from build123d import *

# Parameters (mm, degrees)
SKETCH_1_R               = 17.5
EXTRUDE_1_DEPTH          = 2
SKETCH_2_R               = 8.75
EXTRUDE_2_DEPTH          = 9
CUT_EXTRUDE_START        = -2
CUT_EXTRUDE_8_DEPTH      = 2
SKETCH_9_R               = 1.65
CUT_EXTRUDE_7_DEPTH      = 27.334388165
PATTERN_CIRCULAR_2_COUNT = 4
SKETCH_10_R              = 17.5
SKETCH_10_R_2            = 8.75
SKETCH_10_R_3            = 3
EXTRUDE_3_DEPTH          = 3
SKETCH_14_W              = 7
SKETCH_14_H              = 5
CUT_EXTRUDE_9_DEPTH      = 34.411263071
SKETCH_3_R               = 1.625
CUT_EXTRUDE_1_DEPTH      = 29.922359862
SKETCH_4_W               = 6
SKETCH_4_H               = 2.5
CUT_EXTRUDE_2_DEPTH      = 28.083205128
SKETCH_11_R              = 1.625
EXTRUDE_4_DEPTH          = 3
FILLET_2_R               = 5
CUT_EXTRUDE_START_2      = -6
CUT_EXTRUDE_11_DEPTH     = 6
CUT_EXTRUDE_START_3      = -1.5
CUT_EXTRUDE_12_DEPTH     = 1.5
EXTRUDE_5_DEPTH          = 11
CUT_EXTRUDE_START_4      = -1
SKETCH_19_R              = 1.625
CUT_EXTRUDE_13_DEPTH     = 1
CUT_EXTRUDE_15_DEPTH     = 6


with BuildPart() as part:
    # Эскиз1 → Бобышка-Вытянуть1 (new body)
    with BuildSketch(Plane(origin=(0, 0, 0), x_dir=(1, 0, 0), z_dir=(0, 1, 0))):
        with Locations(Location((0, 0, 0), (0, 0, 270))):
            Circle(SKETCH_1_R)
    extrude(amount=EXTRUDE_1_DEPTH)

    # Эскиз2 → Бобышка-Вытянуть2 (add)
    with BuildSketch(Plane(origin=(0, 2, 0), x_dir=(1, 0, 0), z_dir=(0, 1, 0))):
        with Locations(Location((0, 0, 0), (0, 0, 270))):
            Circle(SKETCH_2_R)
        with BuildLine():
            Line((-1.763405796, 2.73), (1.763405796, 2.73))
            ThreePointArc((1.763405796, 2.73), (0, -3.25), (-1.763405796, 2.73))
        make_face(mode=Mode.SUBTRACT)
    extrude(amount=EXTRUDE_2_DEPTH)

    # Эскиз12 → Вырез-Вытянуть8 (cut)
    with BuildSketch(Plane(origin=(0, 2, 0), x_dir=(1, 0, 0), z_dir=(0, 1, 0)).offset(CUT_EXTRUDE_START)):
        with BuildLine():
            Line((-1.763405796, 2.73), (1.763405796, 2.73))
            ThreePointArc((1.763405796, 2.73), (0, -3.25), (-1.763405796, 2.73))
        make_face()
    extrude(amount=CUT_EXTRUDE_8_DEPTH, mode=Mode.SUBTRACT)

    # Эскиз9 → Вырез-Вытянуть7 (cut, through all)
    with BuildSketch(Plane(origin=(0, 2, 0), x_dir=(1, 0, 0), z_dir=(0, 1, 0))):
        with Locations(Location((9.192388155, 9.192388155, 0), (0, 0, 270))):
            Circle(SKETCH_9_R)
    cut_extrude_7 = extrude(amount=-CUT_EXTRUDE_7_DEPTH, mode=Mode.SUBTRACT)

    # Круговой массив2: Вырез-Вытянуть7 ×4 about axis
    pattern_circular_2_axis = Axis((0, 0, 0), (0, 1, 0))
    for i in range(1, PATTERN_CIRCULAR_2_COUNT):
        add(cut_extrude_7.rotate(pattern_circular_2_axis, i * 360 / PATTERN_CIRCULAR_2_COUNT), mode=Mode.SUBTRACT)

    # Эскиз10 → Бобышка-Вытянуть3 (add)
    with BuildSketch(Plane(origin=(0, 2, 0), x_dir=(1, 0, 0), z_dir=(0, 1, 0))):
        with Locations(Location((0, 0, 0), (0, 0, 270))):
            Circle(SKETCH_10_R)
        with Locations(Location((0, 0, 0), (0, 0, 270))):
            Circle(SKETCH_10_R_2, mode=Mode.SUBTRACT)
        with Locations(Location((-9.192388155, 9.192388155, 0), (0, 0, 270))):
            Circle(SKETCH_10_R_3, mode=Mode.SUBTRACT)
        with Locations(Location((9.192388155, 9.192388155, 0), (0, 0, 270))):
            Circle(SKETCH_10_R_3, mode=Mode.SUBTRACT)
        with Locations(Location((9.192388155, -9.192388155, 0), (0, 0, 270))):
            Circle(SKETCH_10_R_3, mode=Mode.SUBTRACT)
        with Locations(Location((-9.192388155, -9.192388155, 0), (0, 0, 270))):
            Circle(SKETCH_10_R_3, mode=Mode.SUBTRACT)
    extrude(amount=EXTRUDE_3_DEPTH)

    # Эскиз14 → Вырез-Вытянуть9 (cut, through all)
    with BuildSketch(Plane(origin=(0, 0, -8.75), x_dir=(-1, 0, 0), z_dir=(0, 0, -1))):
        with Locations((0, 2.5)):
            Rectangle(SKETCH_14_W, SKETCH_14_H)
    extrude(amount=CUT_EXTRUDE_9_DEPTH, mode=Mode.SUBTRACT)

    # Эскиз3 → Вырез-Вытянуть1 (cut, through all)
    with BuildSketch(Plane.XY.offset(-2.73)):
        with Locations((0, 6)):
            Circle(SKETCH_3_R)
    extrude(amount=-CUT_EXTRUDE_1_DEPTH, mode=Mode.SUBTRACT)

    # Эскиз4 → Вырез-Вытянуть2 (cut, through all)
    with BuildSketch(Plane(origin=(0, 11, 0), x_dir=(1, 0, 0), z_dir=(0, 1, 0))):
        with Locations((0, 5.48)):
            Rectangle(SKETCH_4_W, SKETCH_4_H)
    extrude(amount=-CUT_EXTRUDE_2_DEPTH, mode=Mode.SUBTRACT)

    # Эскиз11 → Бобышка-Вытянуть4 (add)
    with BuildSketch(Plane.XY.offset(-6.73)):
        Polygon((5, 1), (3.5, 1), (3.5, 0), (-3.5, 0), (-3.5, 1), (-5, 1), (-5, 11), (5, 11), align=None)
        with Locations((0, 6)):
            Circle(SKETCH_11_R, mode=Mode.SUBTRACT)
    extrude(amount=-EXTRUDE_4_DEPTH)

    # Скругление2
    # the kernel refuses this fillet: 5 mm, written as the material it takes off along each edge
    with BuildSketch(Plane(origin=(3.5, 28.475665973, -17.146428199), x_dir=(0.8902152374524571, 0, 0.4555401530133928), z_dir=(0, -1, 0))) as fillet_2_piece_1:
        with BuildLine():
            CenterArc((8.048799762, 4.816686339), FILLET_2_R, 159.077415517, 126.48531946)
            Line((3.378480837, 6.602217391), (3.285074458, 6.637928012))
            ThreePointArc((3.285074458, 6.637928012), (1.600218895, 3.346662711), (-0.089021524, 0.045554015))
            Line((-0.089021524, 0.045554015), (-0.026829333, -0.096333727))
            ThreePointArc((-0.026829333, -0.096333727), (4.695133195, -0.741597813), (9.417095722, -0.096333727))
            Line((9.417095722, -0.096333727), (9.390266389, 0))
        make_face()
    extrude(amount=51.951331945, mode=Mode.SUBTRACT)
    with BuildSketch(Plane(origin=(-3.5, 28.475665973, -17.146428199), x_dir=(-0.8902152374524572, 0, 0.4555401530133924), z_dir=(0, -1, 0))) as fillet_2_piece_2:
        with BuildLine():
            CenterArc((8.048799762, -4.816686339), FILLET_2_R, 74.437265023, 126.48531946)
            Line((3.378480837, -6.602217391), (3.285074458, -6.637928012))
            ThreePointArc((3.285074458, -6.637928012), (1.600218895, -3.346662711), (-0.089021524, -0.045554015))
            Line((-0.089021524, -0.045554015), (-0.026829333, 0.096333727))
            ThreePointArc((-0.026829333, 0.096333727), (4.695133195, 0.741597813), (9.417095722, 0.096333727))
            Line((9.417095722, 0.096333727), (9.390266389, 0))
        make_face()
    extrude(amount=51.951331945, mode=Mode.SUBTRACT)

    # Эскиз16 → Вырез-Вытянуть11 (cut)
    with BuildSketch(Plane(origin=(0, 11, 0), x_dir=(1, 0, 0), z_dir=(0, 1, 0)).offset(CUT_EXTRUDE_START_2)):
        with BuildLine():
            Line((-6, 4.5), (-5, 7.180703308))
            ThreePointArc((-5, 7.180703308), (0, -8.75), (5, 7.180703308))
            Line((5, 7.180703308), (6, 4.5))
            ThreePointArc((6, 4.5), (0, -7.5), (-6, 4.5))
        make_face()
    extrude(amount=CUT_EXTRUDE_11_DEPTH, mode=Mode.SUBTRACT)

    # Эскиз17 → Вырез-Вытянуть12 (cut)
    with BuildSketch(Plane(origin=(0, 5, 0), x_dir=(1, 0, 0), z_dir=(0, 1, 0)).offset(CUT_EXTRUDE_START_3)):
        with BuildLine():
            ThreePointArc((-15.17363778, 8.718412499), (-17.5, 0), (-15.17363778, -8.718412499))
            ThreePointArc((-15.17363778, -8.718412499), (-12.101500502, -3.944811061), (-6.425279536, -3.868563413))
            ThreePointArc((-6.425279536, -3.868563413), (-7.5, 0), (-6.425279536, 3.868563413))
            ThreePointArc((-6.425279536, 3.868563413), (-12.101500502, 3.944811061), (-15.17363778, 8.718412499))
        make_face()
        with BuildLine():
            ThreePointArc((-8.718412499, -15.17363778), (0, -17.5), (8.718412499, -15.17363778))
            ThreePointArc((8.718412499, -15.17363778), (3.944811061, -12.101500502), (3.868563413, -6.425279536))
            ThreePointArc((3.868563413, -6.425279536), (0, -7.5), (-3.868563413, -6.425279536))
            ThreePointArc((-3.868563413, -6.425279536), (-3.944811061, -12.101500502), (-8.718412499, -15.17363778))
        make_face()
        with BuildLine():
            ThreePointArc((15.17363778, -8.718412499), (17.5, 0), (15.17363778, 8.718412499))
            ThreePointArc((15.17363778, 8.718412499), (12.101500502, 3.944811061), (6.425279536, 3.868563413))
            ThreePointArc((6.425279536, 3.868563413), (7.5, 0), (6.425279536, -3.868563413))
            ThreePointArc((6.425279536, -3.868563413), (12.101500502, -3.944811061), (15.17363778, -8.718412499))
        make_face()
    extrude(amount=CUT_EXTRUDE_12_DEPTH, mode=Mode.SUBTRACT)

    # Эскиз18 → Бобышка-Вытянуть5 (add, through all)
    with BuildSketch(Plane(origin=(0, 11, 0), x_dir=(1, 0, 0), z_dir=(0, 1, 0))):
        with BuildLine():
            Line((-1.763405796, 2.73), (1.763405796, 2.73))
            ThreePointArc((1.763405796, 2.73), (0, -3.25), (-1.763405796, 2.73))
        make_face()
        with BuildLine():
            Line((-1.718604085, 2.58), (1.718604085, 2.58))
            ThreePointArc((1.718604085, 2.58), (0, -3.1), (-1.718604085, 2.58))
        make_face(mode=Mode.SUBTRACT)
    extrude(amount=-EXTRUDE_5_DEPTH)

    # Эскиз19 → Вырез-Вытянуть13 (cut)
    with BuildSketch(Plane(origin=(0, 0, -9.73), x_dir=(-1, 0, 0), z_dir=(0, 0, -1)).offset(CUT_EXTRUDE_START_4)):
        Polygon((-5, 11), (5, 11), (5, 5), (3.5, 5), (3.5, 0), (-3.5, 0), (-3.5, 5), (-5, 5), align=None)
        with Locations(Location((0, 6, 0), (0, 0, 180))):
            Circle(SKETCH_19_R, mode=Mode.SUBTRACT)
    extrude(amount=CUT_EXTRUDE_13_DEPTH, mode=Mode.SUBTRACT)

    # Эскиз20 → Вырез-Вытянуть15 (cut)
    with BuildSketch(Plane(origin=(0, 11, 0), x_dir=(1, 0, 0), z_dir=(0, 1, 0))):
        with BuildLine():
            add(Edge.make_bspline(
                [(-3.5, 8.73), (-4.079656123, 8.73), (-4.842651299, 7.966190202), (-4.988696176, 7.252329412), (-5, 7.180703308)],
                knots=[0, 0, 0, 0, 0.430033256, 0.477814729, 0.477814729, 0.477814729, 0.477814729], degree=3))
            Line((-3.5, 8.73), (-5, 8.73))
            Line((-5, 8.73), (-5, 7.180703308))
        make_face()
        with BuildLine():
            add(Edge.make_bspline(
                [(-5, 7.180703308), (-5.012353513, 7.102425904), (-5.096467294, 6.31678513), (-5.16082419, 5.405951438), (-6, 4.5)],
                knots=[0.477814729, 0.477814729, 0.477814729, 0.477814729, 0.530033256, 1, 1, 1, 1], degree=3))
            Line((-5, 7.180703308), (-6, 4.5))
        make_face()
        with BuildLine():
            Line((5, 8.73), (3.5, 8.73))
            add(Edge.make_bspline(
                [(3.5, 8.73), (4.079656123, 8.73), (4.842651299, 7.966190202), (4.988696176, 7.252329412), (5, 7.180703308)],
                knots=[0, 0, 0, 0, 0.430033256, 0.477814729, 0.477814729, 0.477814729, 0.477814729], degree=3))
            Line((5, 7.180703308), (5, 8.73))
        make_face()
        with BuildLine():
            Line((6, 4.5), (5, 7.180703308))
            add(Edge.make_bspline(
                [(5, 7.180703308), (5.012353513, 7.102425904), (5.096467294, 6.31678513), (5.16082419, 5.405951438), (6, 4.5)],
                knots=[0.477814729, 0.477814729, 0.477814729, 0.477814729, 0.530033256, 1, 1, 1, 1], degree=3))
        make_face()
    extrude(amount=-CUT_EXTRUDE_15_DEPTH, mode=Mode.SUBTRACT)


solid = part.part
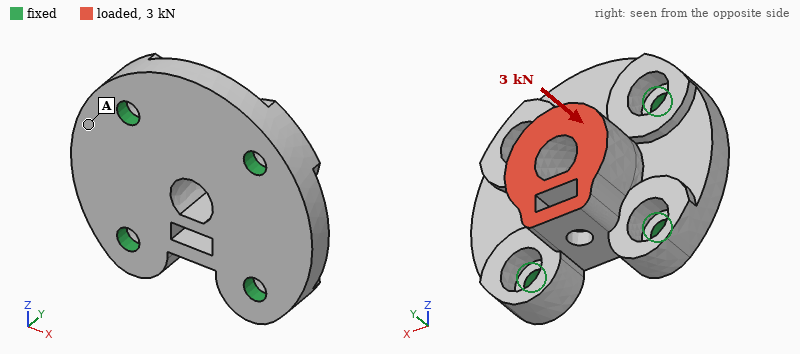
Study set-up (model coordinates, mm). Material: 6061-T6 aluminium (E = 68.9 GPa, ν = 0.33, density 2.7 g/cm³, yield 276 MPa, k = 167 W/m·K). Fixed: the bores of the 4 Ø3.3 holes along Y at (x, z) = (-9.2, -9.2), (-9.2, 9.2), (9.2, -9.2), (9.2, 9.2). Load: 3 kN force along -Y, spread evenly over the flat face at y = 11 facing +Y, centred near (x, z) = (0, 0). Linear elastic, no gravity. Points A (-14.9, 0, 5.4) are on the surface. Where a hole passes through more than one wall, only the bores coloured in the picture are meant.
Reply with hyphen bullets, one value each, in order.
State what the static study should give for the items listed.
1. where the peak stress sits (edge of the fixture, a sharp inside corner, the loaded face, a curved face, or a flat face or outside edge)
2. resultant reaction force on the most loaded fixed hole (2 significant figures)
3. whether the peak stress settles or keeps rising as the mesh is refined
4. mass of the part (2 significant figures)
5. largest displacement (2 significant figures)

- edge of the fixture
- 940 N
- keeps rising
- 11 g
- 15 µm
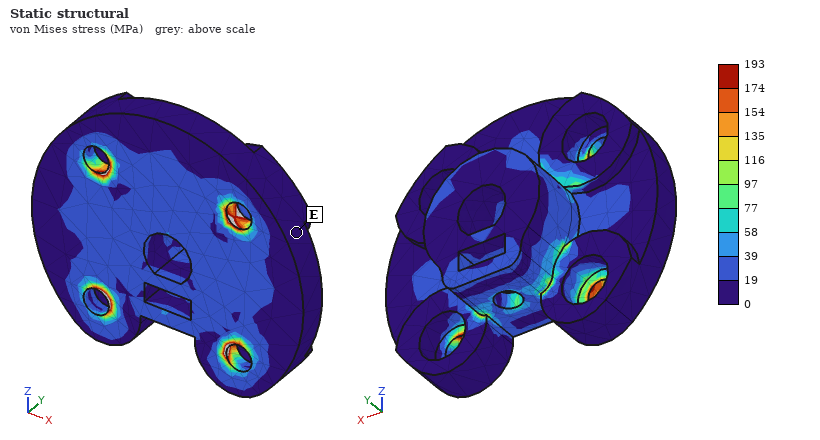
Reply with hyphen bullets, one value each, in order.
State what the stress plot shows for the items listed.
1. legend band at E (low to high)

- 0 to 19 MPa
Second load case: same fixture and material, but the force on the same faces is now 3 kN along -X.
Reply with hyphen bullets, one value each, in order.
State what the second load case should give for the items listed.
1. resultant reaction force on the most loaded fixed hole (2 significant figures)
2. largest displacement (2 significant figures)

- 1.3 kN
- 36 µm
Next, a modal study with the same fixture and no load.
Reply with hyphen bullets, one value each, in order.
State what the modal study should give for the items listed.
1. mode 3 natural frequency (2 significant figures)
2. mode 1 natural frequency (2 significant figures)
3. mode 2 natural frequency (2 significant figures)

- 31 kHz
- 30 kHz
- 30 kHz
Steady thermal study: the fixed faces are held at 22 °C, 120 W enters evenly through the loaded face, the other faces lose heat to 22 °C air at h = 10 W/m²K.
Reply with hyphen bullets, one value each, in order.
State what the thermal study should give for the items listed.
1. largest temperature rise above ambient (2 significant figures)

- 72 K
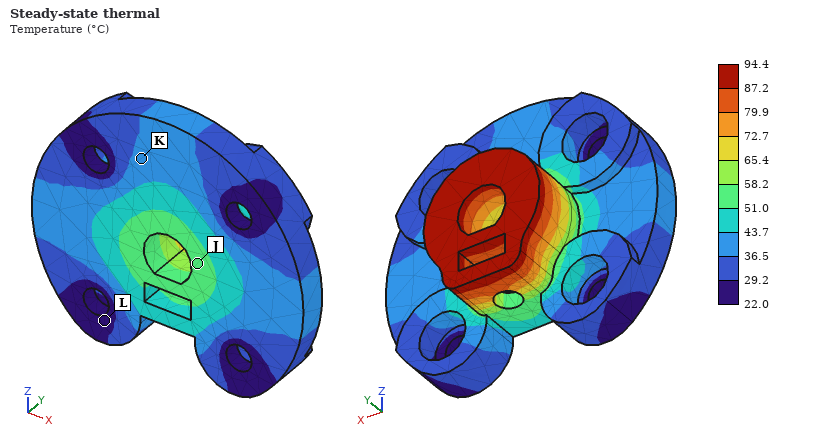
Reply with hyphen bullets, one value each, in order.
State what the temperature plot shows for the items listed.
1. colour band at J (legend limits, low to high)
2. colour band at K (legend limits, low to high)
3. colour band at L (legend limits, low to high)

- 51.0 to 58.2 °C
- 36.5 to 43.7 °C
- 22.0 to 29.2 °C
